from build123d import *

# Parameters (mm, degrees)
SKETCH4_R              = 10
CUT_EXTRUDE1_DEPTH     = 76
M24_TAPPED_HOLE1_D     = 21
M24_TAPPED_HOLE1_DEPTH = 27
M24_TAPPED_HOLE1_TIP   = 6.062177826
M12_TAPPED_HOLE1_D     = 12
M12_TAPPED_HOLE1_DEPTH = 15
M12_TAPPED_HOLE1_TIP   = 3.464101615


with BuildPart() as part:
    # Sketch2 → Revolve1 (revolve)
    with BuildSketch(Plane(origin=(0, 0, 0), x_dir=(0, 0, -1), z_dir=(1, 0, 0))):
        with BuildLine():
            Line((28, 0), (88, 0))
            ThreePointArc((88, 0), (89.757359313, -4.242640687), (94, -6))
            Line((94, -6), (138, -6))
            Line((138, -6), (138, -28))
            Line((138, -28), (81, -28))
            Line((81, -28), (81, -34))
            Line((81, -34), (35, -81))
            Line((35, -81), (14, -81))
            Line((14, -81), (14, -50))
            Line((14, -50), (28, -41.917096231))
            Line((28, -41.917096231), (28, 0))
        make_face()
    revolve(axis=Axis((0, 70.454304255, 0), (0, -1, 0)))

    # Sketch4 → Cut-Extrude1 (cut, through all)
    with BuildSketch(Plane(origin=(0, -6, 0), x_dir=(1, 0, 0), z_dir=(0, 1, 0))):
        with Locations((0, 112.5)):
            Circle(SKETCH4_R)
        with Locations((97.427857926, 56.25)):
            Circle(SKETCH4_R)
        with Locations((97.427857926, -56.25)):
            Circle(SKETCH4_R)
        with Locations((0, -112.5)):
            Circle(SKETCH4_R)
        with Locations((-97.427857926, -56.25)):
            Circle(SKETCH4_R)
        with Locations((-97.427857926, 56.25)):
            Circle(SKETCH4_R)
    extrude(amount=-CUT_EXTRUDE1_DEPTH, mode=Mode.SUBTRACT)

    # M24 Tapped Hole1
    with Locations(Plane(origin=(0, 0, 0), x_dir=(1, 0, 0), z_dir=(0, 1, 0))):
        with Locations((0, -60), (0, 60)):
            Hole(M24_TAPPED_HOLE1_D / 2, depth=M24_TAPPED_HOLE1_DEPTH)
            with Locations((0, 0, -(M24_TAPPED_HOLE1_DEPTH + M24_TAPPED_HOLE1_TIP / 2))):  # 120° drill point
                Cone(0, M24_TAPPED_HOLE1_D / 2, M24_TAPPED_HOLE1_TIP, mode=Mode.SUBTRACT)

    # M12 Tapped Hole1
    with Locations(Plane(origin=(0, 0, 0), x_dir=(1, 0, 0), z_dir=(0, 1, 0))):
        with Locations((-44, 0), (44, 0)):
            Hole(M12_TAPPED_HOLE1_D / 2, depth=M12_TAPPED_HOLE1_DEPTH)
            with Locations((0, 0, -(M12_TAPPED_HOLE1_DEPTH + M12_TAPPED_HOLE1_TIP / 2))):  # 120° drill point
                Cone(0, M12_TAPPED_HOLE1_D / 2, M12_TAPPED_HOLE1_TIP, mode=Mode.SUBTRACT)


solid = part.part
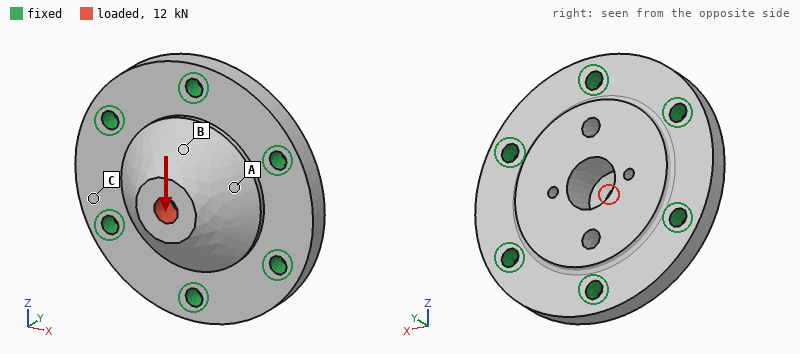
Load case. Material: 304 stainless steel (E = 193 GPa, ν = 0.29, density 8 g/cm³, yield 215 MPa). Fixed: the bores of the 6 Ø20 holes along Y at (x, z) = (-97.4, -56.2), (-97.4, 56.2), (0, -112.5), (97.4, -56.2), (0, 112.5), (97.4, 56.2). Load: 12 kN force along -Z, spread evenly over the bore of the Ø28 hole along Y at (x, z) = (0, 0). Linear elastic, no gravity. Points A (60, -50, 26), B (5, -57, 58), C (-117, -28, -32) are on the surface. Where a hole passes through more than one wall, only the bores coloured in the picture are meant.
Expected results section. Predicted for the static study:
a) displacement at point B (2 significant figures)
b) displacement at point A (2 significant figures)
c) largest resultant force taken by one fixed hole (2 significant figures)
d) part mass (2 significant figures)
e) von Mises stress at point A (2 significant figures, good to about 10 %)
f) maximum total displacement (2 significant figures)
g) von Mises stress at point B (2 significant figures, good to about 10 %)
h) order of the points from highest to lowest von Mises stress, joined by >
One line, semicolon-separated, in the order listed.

1.8 µm; 1.1 µm; 3.4 kN; 15 kg; 1.5 MPa; 2.8 µm; 2.9 MPa; B > A > C
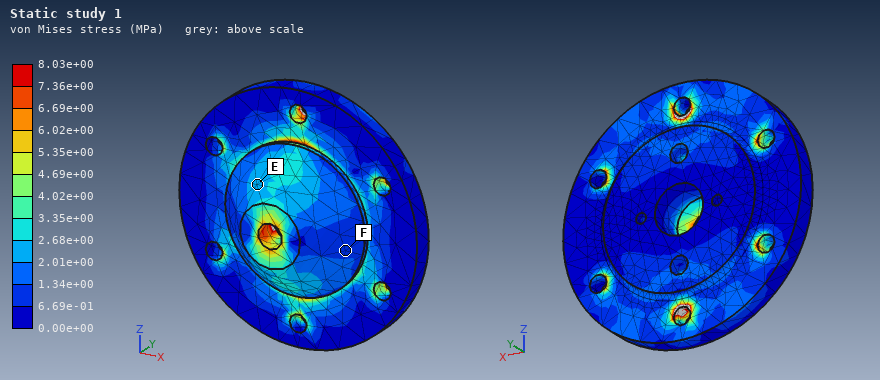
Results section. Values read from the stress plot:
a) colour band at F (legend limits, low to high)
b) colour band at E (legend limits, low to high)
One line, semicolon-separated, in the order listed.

6.69e-01 to 1.34e+00 MPa; 2.01e+00 to 2.68e+00 MPa
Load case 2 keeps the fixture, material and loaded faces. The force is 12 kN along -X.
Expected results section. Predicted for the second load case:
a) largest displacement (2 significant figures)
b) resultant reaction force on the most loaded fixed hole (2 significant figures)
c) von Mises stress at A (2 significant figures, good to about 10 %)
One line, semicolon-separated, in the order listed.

2.8 µm; 3.1 kN; 2.6 MPa
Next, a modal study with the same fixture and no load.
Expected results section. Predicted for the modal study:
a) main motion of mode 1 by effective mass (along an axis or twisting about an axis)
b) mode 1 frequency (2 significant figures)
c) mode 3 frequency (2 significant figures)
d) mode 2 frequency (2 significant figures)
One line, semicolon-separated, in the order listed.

along Y; 4200 Hz; 5900 Hz; 5900 Hz
